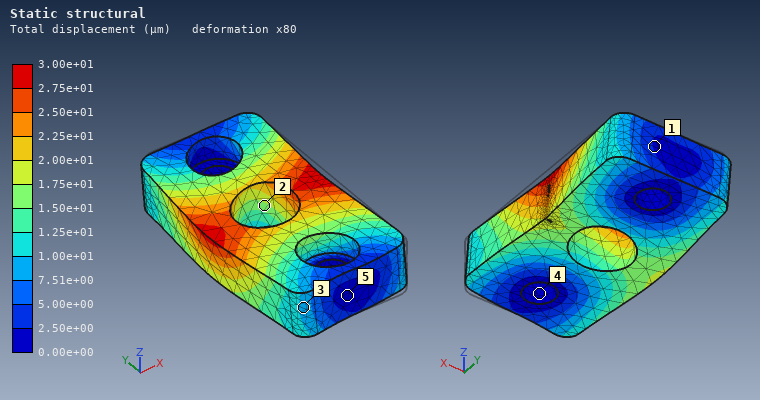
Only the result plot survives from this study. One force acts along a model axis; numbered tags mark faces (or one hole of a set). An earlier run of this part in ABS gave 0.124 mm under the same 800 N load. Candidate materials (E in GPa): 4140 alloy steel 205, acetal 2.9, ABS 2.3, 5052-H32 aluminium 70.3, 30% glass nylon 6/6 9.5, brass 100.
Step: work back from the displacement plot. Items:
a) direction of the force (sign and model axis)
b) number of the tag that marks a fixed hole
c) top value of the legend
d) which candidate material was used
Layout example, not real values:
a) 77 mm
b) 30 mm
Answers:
a) -X
b) 4
c) 3.00e+01 µm
d) 30% glass nylon 6/6
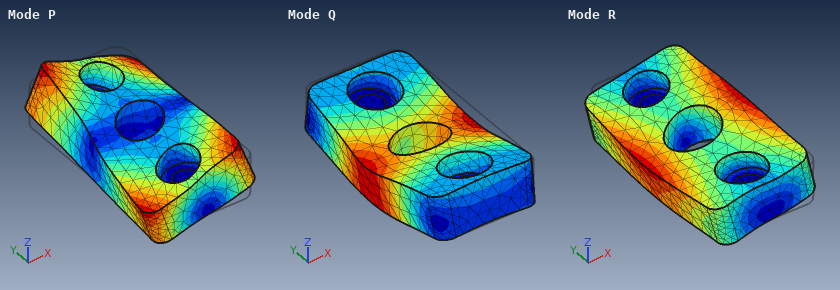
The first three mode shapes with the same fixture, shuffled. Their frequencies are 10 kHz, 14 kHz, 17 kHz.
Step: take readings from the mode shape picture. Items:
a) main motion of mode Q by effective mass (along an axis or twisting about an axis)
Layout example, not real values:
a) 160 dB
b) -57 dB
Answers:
a) along Z
